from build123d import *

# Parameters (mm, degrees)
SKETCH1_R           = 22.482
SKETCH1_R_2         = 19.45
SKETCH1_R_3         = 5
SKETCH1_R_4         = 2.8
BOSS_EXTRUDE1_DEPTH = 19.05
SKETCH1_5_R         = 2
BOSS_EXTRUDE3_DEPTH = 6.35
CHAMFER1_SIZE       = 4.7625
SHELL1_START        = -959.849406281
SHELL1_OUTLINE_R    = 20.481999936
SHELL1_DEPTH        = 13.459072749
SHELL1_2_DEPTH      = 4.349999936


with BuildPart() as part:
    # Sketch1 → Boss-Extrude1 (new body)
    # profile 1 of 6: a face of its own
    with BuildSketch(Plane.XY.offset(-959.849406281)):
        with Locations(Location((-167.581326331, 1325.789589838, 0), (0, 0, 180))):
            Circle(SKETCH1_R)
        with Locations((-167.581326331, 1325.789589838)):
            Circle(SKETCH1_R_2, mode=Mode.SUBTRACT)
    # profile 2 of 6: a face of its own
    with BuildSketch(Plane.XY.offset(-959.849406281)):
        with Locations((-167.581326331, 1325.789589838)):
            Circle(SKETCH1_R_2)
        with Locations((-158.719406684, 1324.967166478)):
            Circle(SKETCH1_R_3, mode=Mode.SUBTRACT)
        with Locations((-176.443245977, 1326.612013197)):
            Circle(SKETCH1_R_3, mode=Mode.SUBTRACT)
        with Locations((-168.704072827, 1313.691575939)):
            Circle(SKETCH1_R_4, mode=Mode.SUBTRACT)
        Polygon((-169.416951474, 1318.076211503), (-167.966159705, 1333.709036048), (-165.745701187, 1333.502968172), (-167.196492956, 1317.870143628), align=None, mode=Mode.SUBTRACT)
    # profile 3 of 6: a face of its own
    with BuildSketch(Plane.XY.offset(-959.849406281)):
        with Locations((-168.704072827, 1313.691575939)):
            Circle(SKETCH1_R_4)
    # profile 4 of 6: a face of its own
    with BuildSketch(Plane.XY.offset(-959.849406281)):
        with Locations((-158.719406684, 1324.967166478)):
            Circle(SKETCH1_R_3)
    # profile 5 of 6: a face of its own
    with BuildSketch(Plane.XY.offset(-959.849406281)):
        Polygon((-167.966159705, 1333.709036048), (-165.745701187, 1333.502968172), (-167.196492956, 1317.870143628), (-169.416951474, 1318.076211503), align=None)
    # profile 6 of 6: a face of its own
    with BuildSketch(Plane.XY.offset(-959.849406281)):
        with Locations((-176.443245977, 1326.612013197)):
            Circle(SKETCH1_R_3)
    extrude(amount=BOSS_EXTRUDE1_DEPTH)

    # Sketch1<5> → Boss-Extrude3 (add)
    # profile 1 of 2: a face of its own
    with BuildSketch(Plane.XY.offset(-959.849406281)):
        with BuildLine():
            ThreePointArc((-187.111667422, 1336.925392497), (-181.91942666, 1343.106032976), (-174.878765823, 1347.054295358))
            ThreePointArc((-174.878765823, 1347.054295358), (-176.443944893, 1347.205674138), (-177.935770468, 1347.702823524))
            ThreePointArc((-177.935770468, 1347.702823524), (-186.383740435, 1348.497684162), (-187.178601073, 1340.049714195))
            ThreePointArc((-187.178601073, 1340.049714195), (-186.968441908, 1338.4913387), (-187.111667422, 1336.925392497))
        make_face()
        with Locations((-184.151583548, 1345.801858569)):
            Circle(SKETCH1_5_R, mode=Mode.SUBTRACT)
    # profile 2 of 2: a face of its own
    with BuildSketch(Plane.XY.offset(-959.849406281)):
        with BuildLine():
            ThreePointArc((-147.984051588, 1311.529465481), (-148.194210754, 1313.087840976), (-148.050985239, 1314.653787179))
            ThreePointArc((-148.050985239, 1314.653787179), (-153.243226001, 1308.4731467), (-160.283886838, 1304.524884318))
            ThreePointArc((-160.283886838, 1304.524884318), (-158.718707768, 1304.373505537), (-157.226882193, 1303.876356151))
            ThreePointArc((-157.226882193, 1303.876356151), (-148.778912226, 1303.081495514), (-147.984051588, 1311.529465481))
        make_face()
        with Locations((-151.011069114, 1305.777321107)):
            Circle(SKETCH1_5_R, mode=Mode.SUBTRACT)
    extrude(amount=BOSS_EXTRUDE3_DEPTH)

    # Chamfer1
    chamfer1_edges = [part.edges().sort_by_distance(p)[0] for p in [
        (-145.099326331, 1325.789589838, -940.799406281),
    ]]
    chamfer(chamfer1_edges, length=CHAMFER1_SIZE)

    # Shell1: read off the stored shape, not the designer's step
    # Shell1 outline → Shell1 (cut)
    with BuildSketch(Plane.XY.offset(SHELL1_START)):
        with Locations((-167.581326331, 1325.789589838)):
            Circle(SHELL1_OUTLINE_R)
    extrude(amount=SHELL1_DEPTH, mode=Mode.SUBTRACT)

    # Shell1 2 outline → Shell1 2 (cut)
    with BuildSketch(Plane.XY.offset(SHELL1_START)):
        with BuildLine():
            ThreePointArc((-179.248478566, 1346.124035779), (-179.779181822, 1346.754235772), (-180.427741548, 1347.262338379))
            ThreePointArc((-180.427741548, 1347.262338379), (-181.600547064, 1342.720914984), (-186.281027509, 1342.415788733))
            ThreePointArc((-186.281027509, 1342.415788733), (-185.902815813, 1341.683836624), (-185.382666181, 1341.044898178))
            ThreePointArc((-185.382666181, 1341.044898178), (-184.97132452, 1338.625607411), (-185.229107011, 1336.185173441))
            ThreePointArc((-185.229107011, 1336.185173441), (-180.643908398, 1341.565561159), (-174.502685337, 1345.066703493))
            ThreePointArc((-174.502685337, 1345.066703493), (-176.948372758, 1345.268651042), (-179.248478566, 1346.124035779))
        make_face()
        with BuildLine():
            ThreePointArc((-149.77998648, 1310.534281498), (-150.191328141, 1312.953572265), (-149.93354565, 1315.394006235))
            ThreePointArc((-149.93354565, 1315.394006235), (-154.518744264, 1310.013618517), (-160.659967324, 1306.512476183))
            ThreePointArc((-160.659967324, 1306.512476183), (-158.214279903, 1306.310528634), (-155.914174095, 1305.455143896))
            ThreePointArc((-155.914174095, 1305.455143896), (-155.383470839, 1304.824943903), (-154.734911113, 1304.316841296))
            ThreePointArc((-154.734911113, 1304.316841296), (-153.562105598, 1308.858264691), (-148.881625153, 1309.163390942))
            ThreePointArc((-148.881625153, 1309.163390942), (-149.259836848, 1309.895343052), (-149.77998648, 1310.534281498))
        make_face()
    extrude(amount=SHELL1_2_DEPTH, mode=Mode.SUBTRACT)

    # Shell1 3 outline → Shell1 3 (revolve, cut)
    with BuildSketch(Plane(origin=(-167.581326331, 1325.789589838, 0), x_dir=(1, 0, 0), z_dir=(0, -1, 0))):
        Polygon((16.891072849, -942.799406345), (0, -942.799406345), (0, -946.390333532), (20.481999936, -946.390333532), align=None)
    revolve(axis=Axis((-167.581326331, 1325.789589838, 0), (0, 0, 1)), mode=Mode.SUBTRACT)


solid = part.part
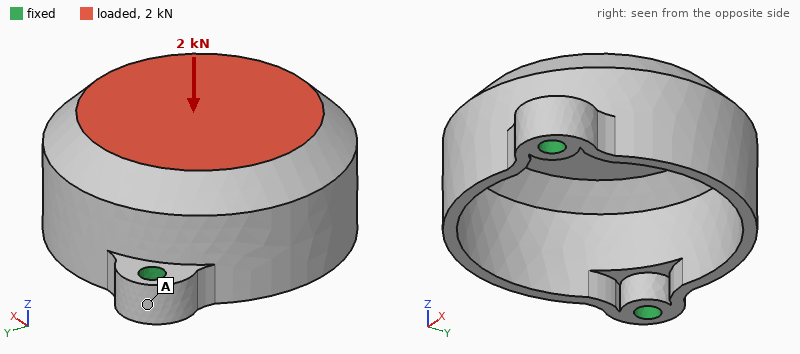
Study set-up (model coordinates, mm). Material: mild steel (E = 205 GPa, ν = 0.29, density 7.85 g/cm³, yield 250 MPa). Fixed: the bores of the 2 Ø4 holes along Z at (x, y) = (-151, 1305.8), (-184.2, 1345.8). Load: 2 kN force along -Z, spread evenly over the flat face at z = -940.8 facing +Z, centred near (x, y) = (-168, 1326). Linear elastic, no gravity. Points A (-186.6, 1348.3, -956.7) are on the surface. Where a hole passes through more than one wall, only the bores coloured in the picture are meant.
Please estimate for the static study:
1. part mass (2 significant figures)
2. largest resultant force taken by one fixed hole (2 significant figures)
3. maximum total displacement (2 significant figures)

60 g
1.2 kN
43 µm
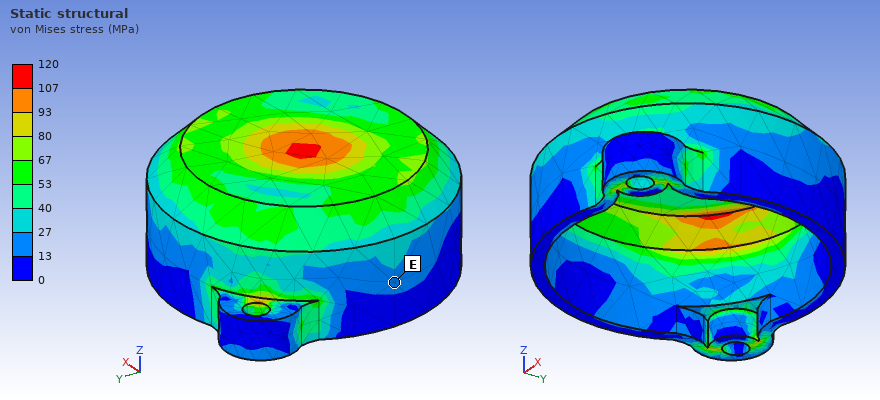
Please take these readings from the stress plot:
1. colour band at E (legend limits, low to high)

13 to 27 MPa
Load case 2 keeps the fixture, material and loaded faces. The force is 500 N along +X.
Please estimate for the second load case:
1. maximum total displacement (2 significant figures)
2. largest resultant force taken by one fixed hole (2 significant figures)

13 µm
270 N
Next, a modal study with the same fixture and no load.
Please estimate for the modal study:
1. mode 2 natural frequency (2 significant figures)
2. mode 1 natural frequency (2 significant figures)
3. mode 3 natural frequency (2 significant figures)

6500 Hz
4300 Hz
7300 Hz
